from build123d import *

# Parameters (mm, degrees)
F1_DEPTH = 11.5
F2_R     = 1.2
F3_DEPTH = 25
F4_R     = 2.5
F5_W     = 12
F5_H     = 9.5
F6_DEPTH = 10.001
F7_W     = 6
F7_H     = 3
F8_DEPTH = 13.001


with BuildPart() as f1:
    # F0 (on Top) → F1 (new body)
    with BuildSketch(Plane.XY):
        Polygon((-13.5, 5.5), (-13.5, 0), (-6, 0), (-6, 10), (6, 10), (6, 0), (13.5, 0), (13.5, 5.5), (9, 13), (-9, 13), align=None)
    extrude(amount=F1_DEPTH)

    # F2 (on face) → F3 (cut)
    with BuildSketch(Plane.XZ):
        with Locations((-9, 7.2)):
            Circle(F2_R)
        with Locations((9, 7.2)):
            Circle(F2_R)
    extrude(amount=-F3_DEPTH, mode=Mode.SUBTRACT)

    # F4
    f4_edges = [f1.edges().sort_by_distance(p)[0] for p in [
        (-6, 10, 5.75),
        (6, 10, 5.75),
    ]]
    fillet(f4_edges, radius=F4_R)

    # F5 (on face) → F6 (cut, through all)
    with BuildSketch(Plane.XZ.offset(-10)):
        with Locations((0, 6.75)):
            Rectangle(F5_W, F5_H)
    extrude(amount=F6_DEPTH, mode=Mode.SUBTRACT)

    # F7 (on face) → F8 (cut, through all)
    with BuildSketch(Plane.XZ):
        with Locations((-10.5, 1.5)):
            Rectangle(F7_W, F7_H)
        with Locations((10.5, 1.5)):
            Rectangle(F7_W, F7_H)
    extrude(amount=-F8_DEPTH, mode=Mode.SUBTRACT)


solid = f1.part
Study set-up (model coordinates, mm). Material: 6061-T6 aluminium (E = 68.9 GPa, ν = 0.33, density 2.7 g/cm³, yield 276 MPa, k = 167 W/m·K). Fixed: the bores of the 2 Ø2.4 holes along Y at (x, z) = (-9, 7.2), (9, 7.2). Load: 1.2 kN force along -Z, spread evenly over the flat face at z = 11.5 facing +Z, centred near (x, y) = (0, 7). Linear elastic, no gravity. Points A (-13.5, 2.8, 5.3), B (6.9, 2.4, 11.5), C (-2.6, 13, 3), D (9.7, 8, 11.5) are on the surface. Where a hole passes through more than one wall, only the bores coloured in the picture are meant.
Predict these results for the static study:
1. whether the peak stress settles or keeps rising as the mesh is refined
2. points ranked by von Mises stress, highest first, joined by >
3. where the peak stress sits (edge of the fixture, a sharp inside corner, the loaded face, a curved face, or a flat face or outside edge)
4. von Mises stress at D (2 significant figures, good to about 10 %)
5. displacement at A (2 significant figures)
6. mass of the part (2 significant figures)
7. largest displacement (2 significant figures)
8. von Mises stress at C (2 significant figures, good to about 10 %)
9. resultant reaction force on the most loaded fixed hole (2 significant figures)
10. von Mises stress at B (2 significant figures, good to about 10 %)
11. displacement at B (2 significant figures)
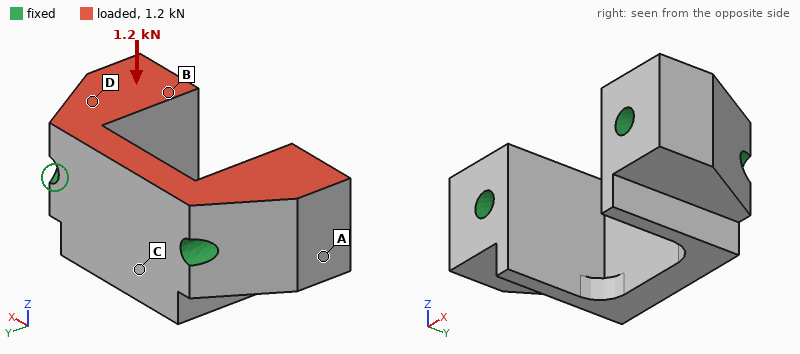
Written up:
keeps rising
D > B > C > A
edge of the fixture
9.3 MPa
0.35 µm
4.8 g
1.6 µm
4.3 MPa
600 N
6.5 MPa
0.35 µm
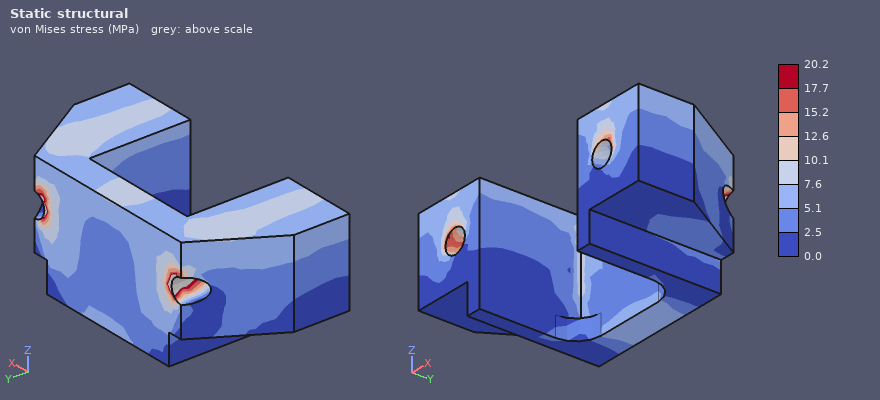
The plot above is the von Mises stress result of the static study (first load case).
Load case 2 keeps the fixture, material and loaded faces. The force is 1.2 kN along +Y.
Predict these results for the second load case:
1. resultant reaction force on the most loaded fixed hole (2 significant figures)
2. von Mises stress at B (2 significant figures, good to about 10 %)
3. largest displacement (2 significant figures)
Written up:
600 N
13 MPa
8.2 µm
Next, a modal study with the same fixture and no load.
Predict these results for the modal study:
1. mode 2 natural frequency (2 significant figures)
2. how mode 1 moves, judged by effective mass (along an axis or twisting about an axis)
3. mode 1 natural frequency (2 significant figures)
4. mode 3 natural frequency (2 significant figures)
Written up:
64 kHz
along Y
53 kHz
70 kHz
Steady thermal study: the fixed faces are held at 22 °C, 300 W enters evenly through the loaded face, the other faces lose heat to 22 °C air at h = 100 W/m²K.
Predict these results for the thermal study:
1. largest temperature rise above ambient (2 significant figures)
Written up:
65 K
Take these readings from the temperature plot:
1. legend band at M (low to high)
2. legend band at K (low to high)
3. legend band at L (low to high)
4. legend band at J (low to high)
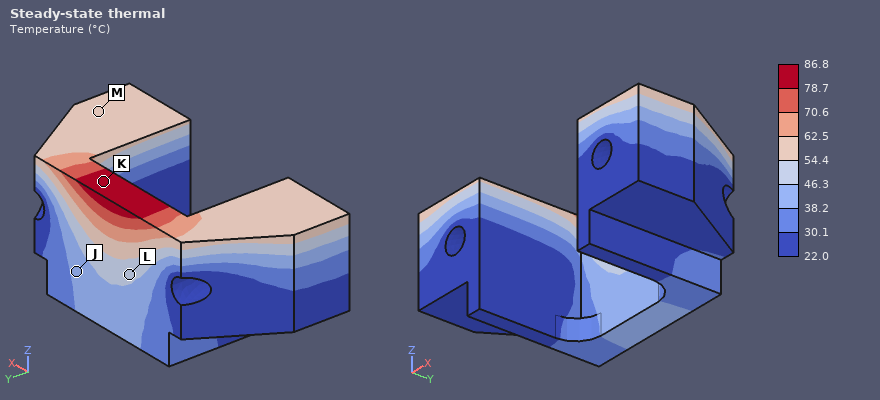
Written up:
54.4 to 62.5 °C
78.7 to 86.8 °C
46.3 to 54.4 °C
38.2 to 46.3 °C
